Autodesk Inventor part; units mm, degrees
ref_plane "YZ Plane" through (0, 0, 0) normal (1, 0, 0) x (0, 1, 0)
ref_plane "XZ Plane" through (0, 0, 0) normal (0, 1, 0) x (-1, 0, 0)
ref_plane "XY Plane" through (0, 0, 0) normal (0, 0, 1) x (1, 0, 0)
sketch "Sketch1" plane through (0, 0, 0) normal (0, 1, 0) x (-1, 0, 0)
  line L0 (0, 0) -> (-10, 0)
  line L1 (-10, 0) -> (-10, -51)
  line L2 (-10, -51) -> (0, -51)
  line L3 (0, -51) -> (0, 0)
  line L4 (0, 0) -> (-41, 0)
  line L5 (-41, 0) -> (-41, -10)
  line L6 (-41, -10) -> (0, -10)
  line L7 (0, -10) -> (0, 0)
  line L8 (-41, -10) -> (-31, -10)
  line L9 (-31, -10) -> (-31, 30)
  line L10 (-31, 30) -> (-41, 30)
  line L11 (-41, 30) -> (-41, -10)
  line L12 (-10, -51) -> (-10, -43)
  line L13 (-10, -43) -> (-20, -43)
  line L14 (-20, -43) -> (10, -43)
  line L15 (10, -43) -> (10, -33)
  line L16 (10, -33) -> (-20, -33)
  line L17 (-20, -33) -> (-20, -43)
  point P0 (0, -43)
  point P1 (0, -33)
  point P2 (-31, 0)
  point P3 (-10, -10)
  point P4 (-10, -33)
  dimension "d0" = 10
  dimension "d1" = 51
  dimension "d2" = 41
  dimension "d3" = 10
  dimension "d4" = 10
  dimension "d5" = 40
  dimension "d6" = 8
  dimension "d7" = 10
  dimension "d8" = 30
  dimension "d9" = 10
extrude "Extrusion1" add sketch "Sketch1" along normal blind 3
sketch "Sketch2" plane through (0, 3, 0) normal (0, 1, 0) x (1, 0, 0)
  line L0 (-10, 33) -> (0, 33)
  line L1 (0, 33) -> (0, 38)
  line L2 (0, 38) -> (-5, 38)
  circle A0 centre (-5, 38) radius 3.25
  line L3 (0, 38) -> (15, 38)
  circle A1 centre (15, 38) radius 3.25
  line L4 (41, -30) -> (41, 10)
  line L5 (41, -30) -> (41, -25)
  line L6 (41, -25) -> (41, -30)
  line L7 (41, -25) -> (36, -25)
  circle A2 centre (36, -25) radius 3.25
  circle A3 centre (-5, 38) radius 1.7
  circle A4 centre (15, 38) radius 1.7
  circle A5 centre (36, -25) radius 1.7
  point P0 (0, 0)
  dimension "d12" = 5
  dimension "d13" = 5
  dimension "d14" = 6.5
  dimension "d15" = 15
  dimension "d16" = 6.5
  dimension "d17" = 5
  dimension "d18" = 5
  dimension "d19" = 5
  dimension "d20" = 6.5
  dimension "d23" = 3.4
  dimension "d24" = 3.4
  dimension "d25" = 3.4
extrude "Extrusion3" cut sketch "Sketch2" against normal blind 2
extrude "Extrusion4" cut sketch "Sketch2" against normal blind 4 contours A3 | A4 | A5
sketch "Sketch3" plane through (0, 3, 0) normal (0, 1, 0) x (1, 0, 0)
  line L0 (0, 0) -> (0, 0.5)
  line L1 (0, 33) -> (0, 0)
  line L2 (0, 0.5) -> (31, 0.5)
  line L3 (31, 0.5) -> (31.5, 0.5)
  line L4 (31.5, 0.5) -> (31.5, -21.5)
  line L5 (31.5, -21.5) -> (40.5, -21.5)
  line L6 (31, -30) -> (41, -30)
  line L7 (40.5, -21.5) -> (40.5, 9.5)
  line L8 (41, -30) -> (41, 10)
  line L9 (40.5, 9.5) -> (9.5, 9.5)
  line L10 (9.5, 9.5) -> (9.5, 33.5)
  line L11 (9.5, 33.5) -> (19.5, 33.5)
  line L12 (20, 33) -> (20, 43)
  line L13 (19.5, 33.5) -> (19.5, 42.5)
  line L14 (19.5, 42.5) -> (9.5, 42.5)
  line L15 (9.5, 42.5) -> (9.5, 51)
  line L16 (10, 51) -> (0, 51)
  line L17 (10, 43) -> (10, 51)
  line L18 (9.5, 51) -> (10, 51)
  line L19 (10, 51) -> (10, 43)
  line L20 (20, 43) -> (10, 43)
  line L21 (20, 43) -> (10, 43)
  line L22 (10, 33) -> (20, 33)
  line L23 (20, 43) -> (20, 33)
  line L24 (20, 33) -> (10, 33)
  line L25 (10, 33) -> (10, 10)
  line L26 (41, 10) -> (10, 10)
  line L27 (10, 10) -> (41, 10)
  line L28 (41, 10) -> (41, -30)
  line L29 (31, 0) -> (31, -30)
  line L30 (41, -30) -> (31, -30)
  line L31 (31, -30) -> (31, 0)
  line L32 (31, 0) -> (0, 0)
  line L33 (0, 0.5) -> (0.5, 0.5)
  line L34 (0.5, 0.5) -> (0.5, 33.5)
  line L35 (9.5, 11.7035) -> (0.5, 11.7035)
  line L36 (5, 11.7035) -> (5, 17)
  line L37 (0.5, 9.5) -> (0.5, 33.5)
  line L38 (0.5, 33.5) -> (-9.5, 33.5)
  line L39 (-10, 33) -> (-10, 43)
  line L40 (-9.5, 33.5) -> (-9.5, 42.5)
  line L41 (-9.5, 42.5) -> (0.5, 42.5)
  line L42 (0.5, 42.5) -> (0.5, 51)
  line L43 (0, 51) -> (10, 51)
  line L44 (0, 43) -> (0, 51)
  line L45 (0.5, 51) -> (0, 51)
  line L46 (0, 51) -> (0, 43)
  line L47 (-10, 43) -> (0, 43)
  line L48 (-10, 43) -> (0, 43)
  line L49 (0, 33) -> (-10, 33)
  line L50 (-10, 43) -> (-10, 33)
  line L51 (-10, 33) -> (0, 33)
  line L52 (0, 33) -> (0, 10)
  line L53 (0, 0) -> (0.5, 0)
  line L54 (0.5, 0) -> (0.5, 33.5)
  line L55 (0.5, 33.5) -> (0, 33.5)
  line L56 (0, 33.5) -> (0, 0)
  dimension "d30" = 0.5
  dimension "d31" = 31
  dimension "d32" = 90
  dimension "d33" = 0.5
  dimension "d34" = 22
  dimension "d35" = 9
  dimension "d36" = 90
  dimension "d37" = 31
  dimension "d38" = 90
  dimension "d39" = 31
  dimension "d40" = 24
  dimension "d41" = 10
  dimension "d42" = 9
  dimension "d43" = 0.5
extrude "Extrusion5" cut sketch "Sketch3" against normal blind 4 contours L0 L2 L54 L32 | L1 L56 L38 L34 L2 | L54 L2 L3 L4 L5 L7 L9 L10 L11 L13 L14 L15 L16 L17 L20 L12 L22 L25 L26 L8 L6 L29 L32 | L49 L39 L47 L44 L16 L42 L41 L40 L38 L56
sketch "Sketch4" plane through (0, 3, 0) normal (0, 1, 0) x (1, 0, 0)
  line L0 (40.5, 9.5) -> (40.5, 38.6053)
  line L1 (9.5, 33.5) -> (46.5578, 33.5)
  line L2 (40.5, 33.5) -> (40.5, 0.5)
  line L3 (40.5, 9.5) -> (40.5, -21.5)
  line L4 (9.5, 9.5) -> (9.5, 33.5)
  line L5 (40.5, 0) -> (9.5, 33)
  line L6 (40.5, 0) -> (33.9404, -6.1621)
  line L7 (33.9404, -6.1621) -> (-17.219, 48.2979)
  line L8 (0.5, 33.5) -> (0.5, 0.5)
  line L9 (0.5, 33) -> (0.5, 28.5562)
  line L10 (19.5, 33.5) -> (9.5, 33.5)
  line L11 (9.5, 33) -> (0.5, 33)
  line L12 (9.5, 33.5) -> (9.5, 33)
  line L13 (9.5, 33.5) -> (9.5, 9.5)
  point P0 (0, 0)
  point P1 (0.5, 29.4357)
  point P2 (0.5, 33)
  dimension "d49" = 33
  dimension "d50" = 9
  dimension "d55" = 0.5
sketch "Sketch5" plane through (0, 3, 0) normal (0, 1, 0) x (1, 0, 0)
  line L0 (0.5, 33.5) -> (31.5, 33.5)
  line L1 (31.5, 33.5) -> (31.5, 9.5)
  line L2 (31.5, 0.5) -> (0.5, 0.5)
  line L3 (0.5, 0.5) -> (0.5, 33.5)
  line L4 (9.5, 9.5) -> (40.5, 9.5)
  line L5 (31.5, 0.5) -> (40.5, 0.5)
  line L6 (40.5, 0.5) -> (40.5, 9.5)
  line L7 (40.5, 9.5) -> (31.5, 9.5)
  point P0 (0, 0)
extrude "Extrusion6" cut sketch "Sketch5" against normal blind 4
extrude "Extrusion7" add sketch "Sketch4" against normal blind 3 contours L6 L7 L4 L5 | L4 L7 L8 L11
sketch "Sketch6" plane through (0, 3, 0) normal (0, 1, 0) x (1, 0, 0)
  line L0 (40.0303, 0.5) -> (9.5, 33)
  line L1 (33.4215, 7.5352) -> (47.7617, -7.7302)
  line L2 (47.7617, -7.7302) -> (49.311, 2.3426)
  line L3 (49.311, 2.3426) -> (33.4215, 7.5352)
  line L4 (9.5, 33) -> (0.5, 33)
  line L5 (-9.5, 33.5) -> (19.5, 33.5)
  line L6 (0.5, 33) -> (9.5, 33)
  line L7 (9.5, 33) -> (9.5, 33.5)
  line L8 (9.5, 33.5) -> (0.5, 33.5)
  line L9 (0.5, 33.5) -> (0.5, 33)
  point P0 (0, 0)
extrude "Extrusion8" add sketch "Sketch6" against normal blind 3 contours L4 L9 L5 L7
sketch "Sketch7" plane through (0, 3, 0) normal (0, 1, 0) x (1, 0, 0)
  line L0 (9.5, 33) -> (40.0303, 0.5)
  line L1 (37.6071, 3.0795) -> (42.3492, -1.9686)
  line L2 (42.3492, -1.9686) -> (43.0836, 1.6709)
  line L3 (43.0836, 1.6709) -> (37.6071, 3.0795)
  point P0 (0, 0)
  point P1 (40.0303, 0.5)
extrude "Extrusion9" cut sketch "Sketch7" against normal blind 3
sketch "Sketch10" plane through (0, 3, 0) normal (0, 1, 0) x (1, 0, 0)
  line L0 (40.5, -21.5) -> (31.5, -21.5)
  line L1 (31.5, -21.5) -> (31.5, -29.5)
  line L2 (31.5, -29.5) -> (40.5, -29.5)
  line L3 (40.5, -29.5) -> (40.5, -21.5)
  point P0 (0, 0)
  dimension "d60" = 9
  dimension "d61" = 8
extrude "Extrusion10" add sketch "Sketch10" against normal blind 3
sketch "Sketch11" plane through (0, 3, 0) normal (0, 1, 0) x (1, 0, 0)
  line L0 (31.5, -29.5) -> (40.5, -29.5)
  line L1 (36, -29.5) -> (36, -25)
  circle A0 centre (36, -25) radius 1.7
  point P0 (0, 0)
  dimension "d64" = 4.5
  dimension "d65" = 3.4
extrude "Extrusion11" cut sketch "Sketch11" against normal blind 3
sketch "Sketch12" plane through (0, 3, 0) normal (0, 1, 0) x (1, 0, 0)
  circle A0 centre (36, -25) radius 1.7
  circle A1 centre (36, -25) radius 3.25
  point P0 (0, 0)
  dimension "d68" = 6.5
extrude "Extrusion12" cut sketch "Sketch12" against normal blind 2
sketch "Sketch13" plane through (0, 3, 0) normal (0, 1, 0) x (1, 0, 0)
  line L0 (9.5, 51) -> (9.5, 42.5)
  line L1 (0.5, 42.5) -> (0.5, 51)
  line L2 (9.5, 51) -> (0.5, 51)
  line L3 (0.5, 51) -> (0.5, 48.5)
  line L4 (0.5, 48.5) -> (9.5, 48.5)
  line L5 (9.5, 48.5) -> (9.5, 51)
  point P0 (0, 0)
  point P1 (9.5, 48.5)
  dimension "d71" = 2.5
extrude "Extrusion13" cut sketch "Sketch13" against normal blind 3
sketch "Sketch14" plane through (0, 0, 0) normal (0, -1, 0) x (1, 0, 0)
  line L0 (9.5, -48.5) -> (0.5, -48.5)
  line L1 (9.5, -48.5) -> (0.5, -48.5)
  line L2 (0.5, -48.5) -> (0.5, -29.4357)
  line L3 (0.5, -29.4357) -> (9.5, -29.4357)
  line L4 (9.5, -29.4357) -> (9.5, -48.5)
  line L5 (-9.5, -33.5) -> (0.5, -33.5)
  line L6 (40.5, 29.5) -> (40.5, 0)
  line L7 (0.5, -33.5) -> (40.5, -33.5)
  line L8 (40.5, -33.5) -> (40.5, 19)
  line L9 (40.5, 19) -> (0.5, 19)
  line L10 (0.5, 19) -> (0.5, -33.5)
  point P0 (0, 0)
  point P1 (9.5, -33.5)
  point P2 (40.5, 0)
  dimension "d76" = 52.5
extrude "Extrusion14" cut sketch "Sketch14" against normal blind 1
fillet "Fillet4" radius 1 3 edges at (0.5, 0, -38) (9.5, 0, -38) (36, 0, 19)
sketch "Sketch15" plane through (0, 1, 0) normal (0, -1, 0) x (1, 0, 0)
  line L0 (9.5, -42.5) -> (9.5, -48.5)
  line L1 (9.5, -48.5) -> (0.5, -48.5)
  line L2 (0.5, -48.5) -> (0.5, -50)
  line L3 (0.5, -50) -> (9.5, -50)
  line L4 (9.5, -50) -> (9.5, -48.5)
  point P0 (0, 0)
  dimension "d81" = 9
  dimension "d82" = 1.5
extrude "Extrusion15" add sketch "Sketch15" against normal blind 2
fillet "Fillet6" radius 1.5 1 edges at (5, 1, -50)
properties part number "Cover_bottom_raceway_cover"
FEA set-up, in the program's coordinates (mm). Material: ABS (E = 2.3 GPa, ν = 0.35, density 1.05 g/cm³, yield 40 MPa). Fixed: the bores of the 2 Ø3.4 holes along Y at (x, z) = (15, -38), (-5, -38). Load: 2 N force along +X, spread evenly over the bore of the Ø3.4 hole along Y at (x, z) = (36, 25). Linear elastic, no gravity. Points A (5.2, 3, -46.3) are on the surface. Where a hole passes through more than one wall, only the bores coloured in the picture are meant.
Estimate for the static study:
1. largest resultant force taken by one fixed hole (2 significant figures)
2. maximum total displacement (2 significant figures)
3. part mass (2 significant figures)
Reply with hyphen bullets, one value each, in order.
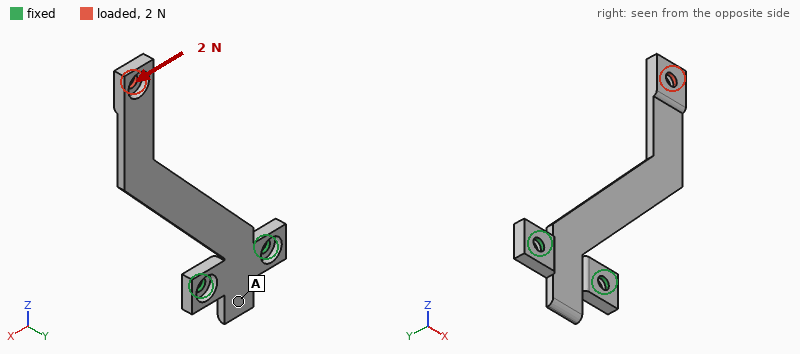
- 7.0 N
- 0.96 mm
- 2.2 g
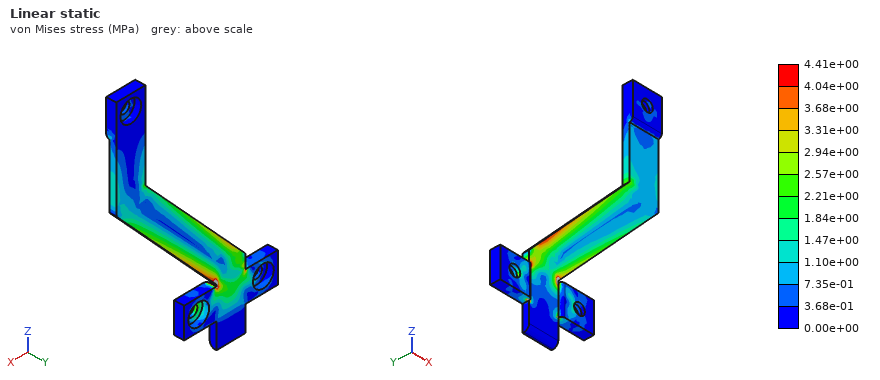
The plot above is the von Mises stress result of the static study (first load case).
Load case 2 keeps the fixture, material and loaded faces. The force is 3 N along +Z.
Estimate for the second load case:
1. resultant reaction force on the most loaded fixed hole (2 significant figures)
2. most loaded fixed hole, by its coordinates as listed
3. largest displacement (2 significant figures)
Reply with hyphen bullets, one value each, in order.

- 6.6 N
- (15, -38)
- 0.97 mm
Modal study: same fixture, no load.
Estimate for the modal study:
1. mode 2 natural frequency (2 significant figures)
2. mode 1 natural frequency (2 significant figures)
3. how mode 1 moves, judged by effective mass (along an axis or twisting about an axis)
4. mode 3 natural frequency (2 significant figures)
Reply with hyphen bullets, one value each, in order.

- 350 Hz
- 82 Hz
- along Y
- 450 Hz
